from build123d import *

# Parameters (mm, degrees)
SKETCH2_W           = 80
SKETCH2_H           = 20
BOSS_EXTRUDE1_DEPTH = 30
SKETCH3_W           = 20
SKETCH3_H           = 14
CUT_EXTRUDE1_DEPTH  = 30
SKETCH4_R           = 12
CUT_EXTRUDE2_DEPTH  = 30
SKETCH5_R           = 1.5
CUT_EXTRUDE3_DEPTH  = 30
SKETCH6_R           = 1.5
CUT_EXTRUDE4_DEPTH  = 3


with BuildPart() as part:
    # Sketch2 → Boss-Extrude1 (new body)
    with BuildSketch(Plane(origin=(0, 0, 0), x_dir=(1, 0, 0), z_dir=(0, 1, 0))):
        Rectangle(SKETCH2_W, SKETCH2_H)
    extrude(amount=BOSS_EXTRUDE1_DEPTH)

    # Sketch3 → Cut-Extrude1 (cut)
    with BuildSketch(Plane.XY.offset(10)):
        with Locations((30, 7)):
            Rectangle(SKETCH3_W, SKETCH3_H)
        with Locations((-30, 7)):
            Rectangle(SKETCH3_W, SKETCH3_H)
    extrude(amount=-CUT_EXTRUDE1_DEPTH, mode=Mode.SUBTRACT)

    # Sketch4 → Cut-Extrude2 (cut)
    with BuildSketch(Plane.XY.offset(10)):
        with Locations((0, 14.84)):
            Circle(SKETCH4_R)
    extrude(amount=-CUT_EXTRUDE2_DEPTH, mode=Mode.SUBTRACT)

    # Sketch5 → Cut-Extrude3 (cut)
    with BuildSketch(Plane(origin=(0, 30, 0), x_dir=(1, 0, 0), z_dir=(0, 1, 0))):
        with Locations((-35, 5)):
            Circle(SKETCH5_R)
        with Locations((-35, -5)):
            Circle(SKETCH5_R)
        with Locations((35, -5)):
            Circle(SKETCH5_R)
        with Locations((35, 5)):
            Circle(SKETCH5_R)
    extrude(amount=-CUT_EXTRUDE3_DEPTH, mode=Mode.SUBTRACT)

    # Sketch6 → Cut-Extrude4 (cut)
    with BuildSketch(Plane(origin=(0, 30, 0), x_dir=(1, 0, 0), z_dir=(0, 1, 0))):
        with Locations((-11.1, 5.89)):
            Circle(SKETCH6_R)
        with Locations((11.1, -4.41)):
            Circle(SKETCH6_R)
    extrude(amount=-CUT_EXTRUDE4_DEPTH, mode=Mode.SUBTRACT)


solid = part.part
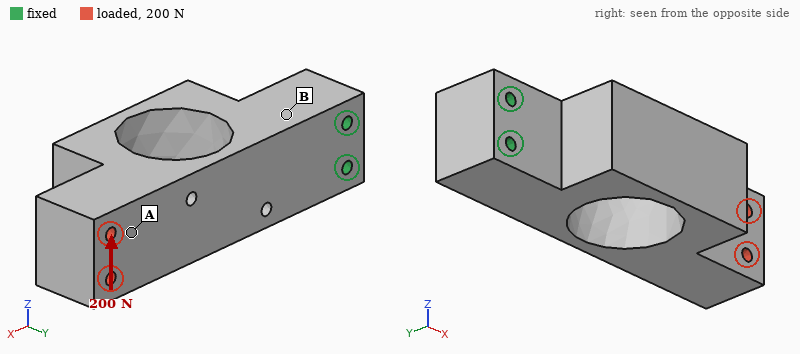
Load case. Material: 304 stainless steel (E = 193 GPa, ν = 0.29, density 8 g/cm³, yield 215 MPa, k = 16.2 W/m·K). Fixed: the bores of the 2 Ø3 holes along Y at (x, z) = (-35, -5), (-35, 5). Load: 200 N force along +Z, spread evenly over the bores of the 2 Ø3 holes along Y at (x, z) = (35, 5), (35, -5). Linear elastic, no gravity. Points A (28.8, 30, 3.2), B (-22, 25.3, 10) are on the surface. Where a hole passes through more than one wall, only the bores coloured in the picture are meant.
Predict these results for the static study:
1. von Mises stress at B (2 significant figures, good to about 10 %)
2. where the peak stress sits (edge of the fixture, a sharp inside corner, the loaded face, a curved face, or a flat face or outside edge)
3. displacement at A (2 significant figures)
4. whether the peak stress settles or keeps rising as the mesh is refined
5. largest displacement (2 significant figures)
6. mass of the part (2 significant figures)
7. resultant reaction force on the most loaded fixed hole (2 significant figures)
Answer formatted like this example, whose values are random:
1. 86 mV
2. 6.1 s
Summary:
1. 11 MPa
2. a sharp inside corner
3. 17 µm
4. keeps rising
5. 22 µm
6. 220 g
7. 1.2 kN
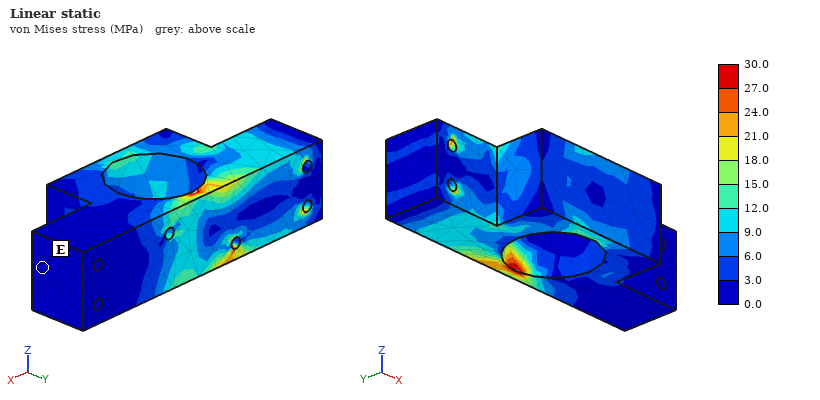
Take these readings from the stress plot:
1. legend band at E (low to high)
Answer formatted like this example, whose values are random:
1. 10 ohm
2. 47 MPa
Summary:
1. 0.0 to 3.0 MPa
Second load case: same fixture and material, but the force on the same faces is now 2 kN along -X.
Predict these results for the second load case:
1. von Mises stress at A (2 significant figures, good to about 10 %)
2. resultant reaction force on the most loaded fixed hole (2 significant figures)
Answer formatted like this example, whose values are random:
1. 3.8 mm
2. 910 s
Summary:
1. 6.4 MPa
2. 1.0 kN
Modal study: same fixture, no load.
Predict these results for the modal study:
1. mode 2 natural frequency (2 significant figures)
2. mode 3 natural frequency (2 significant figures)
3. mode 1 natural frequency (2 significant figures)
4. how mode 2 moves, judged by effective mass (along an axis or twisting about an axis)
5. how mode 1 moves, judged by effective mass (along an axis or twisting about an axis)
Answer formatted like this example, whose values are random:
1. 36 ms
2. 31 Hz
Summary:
1. 2100 Hz
2. 5900 Hz
3. 1800 Hz
4. along Z
5. along Y
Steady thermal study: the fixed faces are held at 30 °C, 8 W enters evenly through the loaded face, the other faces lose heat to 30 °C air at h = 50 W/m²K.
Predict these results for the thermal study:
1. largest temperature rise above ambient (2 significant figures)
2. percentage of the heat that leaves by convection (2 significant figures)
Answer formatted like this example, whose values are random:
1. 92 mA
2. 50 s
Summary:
1. 48 K
2. 87 %
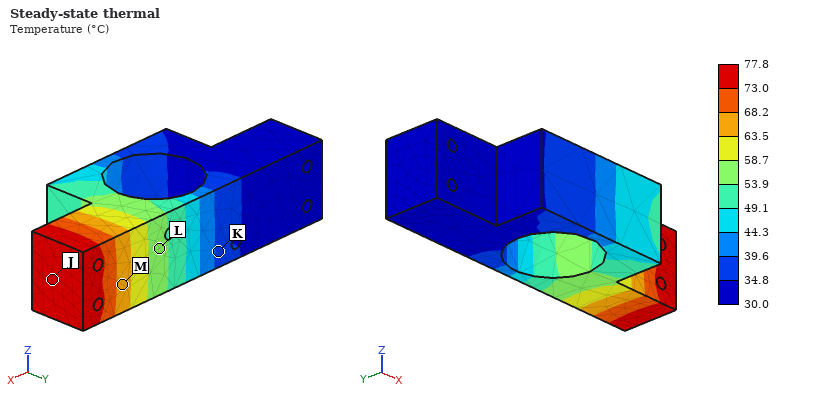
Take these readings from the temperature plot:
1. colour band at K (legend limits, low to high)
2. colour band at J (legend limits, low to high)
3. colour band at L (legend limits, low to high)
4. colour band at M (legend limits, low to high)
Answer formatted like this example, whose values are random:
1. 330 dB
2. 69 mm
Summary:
1. 34.8 to 39.6 °C
2. 73.0 to 77.8 °C
3. 53.9 to 58.7 °C
4. 63.5 to 68.2 °C
